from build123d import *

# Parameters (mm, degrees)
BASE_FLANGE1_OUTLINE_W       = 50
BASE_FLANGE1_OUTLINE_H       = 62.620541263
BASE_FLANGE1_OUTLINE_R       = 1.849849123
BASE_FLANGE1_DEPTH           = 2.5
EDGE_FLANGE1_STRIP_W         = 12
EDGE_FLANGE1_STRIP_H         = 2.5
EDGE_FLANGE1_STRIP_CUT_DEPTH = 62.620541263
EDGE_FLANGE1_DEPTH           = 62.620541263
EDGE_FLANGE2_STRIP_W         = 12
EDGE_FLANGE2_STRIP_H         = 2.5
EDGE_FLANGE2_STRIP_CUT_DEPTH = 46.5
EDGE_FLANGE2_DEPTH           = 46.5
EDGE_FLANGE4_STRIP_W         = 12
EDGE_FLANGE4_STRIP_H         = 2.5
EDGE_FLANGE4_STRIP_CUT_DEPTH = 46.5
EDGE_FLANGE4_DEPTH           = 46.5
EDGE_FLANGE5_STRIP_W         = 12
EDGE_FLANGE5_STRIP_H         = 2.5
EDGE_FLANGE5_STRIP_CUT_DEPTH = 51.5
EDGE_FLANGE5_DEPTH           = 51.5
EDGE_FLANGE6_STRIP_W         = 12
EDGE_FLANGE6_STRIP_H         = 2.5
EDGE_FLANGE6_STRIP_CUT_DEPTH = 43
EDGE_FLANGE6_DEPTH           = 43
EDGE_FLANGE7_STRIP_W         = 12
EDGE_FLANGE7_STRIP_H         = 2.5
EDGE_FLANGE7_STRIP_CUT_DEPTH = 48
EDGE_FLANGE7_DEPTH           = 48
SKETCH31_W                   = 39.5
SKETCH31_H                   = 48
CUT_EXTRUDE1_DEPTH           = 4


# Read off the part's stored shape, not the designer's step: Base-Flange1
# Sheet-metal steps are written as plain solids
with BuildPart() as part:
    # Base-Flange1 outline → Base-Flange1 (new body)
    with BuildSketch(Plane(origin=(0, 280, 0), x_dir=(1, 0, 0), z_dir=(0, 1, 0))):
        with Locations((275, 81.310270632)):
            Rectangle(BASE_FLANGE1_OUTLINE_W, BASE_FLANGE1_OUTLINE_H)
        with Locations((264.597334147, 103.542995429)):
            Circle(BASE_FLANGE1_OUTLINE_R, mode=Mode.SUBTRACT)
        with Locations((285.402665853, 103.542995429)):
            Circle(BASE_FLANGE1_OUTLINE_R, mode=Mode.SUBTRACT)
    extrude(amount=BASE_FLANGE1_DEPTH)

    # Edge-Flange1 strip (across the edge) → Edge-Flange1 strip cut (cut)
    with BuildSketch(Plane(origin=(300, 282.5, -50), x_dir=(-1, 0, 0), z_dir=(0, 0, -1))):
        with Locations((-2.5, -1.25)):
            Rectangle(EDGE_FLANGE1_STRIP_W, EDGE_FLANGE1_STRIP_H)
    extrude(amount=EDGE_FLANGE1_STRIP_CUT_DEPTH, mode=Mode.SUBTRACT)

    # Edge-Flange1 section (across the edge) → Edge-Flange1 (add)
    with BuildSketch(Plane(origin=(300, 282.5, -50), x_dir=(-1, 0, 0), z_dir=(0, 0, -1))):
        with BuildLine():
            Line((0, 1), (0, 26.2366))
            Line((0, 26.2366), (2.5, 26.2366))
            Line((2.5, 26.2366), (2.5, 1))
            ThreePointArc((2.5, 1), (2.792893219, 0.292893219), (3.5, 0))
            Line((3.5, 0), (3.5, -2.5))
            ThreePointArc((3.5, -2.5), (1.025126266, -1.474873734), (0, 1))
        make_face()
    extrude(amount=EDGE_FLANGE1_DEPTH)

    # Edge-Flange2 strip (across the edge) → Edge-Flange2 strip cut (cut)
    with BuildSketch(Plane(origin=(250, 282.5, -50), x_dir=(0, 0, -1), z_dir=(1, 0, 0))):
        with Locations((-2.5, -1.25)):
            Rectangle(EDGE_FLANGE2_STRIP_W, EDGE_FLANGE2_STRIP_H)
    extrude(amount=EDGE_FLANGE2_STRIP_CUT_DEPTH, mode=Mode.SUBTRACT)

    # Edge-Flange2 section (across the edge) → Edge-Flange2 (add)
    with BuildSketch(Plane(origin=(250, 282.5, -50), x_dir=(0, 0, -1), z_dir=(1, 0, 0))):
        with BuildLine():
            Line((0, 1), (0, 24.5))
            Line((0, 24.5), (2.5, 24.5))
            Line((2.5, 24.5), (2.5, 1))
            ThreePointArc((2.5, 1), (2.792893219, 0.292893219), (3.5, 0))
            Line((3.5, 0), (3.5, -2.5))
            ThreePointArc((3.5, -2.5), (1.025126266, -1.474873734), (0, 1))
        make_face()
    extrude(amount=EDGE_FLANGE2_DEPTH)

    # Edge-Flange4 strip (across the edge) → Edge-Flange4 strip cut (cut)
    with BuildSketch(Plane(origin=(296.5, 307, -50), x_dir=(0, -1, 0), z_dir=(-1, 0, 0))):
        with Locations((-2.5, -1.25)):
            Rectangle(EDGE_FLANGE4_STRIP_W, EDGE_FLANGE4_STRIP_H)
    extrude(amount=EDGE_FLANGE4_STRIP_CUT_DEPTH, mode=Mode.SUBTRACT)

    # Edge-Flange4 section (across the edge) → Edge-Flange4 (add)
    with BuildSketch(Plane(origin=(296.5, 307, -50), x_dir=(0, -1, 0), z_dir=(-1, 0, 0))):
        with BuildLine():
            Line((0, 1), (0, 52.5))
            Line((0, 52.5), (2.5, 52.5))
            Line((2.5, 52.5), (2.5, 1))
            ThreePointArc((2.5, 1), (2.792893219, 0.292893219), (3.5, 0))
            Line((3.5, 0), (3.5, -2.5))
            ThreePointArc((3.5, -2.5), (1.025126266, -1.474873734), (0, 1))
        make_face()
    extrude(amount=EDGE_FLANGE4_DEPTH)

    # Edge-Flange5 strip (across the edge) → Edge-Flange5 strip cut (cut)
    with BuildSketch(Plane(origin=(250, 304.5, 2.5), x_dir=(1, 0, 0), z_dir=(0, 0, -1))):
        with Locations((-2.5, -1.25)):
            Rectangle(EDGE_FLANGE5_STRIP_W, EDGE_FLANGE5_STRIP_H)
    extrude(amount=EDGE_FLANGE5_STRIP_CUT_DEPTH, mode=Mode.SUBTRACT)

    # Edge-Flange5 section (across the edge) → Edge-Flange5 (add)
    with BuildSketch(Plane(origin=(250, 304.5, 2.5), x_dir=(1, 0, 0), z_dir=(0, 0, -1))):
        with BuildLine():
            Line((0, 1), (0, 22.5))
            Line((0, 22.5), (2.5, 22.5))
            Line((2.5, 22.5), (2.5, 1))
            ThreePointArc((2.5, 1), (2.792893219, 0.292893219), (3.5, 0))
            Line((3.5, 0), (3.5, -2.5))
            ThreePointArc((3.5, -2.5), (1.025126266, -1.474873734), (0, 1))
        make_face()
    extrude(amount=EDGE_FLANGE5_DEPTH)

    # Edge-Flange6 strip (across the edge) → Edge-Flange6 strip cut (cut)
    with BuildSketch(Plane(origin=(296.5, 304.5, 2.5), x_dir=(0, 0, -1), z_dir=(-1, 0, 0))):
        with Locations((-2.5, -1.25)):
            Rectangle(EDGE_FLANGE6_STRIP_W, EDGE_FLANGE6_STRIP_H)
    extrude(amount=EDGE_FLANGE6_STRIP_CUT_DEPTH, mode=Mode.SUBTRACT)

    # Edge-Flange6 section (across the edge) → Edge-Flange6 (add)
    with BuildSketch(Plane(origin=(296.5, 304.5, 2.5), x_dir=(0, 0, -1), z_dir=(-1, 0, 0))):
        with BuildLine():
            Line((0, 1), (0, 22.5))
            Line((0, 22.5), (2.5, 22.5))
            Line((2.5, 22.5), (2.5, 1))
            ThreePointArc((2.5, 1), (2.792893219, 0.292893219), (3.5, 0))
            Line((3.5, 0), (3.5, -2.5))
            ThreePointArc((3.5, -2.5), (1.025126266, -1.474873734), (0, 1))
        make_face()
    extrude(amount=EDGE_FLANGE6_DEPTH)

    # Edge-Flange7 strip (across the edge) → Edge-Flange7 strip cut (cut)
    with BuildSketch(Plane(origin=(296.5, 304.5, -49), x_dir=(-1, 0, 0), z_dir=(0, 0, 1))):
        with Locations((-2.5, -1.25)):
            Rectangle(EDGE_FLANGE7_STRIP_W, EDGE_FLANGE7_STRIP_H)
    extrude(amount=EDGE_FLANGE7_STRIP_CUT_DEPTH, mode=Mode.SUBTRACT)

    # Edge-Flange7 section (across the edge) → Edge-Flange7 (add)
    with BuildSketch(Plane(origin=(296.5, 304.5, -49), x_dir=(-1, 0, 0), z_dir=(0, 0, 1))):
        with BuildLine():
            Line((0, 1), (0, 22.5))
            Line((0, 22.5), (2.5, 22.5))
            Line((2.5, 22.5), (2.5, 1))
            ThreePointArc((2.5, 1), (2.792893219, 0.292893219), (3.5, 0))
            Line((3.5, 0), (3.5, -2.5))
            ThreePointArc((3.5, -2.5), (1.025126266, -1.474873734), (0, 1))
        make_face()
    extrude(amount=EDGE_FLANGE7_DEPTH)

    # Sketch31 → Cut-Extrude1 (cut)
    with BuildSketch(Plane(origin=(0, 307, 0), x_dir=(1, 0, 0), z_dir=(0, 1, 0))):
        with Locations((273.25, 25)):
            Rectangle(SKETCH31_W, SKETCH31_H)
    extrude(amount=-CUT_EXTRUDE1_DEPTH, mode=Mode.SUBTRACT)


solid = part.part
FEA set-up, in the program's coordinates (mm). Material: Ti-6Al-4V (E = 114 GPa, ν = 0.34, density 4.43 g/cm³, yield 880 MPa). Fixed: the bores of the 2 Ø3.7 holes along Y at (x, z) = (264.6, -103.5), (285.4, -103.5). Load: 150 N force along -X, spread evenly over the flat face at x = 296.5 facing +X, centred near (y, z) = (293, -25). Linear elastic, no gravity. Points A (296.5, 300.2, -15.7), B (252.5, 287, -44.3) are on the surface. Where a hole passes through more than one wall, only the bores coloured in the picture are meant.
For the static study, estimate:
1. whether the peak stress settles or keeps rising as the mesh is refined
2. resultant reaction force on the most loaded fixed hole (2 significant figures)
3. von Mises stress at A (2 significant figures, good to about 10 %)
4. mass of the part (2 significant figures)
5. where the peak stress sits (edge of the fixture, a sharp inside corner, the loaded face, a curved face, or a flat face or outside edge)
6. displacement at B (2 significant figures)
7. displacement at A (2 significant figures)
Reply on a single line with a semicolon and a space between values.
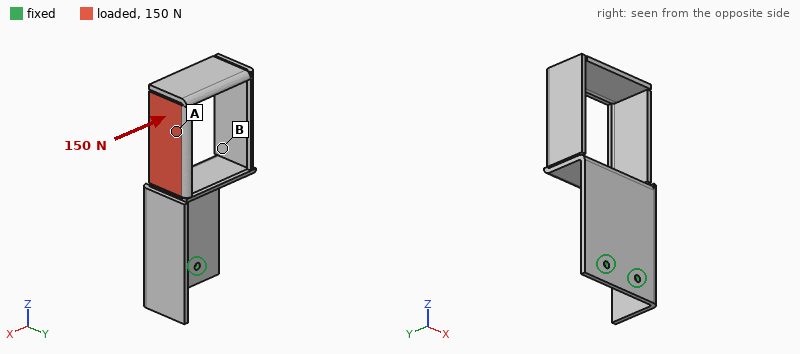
keeps rising; 520 N; 42 MPa; 100 g; a sharp inside corner; 0.21 mm; 0.82 mm
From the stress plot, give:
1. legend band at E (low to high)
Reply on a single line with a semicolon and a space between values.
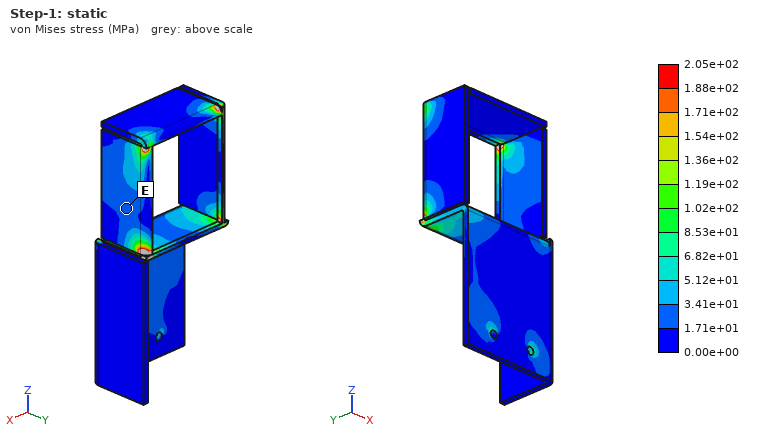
1.71e+01 to 3.41e+01 MPa
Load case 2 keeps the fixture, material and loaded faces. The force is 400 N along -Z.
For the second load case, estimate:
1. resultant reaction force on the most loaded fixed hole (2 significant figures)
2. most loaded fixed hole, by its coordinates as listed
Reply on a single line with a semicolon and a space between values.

570 N; (285.4, -103.5)
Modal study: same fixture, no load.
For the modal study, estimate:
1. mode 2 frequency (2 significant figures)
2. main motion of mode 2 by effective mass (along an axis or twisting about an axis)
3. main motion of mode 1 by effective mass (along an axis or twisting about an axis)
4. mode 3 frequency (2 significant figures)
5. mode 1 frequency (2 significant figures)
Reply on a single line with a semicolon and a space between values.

290 Hz; along X; along Y; 440 Hz; 150 Hz
